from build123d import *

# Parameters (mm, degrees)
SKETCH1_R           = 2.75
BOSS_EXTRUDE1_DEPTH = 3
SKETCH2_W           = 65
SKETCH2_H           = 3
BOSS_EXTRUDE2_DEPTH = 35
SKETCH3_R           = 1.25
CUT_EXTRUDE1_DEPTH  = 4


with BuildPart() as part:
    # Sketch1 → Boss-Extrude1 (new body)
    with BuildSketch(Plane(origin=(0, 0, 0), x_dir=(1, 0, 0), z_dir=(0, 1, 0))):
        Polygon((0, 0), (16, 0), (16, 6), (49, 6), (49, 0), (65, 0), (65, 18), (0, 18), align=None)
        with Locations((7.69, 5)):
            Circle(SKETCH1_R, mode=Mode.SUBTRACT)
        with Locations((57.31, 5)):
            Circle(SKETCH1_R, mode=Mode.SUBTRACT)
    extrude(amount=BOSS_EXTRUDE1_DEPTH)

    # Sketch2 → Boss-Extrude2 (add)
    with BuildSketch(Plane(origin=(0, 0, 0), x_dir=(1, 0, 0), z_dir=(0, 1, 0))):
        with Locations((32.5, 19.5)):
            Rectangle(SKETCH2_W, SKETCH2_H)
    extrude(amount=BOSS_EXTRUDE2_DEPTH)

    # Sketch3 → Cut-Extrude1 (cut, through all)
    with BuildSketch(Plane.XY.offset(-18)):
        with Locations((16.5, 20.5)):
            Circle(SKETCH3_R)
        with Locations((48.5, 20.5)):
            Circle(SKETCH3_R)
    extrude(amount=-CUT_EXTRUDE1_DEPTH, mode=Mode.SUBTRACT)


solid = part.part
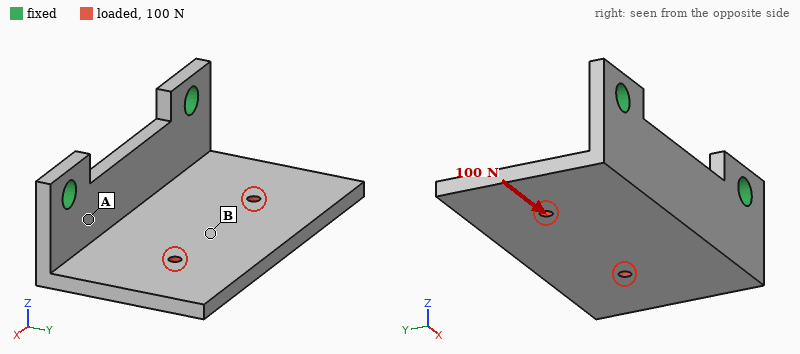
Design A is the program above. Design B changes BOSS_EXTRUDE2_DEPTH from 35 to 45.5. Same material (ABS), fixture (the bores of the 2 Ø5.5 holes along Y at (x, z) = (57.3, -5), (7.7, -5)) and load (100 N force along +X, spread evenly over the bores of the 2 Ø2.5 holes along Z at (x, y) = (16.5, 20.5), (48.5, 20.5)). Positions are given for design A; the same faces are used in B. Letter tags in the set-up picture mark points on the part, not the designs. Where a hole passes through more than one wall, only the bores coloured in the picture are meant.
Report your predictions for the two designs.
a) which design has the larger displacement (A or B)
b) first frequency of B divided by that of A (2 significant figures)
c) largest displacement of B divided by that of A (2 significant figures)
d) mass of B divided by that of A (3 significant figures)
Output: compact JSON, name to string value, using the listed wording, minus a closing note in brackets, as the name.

{"which design has the larger displacement": "B", "first frequency of B divided by that of A": "0.65", "largest displacement of B divided by that of A": "1.1", "mass of B divided by that of A": "1.21"}
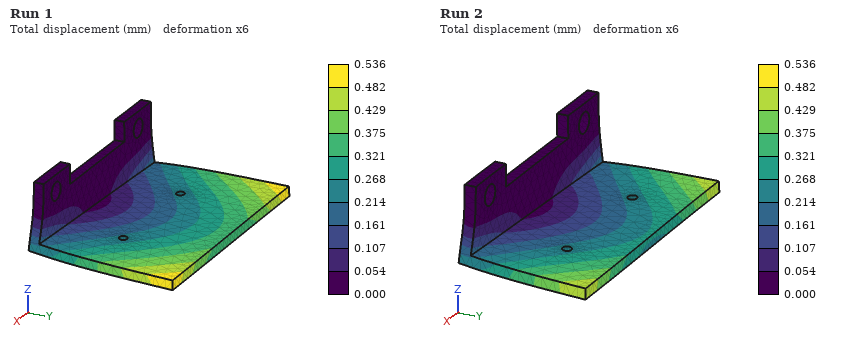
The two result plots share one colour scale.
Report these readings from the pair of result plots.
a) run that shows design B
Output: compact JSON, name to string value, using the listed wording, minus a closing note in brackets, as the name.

{"run that shows design B": "Run 1"}
